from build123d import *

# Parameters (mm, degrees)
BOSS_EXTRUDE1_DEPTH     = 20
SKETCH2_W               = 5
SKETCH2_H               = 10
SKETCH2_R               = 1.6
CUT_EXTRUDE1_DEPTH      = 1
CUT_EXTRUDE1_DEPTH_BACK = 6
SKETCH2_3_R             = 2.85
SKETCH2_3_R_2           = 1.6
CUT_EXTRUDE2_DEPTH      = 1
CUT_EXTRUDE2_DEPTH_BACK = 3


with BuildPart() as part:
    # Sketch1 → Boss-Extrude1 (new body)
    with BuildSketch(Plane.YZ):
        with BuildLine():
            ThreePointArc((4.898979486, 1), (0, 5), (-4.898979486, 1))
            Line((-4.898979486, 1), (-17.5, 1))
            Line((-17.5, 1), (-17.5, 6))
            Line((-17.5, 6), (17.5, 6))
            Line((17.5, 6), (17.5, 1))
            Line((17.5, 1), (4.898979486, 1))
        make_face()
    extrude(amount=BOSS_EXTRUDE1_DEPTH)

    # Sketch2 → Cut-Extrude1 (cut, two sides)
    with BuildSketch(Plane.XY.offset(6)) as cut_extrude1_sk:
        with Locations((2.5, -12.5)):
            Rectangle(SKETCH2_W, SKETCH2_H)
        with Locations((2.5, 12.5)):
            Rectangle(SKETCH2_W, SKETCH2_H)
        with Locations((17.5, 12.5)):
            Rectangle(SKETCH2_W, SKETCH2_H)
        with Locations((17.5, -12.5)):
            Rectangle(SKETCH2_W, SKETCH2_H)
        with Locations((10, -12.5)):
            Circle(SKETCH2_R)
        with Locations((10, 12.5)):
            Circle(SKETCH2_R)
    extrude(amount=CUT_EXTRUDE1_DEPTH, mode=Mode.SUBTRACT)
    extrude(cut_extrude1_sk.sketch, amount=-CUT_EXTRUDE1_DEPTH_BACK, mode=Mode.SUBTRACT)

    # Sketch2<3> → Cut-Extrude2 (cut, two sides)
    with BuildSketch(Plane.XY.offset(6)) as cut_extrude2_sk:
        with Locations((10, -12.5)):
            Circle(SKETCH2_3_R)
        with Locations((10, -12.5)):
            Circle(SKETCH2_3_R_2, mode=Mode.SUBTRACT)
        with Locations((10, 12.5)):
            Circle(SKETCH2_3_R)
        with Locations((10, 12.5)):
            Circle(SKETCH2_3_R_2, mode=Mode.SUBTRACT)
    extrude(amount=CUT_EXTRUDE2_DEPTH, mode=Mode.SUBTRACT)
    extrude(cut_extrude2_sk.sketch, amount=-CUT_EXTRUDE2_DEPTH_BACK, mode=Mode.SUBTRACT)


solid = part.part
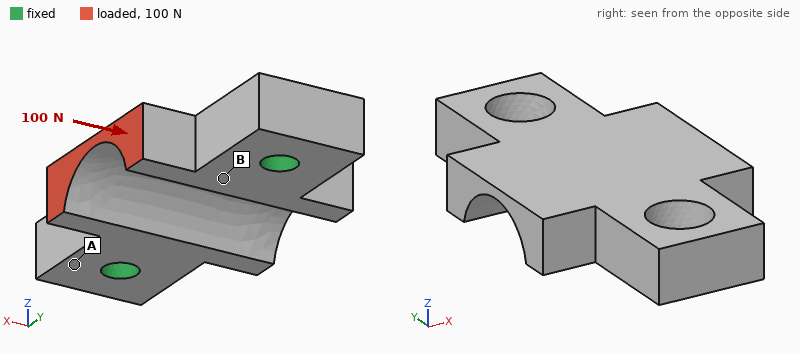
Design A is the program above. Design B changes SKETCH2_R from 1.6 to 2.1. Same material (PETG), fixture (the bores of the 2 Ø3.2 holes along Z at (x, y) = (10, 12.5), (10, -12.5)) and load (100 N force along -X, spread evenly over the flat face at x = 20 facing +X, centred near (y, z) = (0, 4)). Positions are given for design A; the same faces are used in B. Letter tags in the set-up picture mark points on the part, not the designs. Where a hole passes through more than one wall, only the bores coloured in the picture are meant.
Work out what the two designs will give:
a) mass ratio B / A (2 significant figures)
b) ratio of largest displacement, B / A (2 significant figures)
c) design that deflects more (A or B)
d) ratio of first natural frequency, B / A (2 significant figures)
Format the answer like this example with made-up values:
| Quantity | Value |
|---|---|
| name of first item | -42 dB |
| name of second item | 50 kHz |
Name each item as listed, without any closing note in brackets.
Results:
| Quantity | Value |
|---|---|
| mass ratio B / A | 0.99 |
| ratio of largest displacement, B / A | 0.76 |
| design that deflects more | A |
| ratio of first natural frequency, B / A | 1.2 |
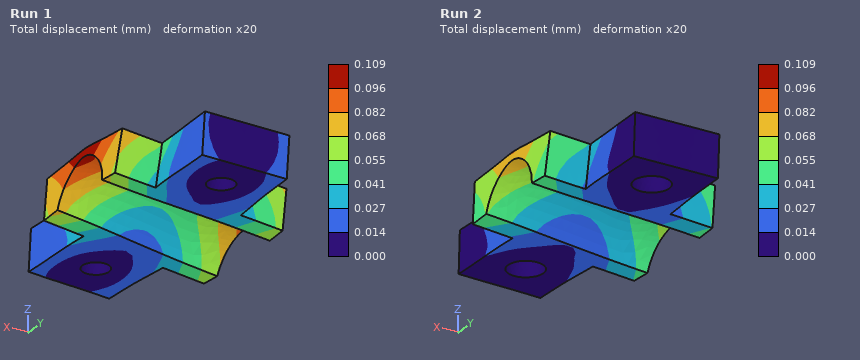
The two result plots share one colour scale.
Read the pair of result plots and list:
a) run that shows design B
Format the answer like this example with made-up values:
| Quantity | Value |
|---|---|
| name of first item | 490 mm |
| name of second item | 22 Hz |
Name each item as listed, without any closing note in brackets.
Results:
| Quantity | Value |
|---|---|
| run that shows design B | Run 2 |
